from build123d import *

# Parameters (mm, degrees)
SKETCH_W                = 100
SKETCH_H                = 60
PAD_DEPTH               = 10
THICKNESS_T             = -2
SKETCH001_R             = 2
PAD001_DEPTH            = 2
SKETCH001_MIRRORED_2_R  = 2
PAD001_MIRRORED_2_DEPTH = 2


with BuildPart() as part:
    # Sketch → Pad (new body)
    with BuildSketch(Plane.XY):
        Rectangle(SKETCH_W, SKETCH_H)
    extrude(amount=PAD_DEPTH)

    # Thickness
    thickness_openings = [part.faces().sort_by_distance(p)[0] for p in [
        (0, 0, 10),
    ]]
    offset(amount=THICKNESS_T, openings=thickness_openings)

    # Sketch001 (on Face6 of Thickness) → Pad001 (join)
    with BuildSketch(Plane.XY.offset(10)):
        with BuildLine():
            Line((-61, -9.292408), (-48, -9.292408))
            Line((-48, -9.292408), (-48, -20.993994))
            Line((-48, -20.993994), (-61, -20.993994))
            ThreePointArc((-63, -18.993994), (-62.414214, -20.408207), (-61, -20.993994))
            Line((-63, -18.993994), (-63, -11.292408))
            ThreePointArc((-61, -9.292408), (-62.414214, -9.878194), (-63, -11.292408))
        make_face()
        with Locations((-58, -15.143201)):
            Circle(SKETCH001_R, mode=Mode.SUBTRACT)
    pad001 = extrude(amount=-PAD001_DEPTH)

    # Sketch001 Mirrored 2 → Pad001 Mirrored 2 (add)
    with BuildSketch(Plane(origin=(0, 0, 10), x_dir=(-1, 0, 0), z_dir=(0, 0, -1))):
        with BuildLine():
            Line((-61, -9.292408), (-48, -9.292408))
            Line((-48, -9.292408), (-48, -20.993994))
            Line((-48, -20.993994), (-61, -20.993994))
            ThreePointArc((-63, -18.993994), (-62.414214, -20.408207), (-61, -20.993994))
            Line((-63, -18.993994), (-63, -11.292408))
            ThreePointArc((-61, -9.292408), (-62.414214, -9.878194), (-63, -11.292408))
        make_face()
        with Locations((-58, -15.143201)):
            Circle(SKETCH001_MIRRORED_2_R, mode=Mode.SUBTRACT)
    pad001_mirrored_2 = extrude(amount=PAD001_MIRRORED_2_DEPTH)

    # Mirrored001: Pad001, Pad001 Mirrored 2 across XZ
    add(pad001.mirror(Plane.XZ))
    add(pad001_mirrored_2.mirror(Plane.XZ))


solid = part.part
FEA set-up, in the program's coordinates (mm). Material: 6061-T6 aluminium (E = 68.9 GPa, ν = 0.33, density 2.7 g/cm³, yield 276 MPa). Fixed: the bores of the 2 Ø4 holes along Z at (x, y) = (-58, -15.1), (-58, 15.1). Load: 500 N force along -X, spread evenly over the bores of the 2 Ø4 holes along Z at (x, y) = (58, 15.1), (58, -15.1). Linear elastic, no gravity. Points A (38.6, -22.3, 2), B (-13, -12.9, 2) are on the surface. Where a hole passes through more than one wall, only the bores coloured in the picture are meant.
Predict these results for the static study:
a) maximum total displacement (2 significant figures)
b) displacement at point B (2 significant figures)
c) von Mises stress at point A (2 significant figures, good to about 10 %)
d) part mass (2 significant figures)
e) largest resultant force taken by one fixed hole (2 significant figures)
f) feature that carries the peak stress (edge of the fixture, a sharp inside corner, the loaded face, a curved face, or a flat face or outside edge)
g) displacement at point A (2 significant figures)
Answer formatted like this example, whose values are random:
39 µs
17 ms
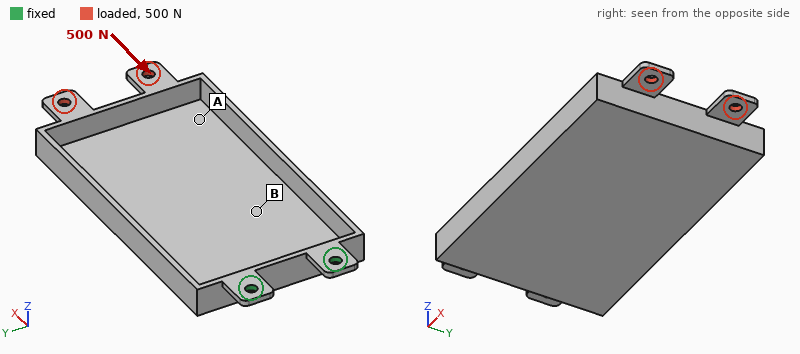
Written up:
1.5 mm
0.30 mm
18 MPa
49 g
250 N
a flat face or outside edge
0.94 mm
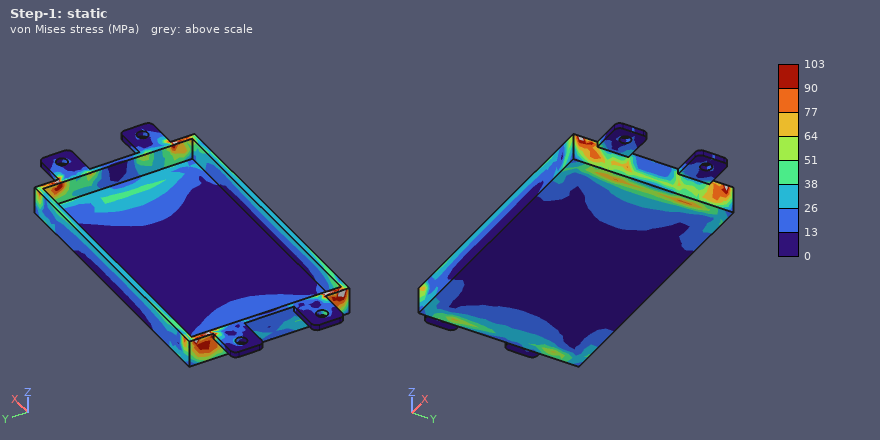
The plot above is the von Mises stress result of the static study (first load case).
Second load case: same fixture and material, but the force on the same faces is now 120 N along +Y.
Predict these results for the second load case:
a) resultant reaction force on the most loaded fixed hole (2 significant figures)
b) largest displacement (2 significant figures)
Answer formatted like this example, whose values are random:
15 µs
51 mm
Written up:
350 N
1.2 mm
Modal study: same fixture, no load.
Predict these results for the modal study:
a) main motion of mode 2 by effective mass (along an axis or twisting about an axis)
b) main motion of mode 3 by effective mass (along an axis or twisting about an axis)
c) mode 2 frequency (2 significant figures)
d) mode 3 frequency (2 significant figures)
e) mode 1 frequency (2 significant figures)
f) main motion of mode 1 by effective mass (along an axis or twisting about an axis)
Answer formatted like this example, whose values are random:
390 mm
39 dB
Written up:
along Y
along Y
400 Hz
900 Hz
110 Hz
along Z
